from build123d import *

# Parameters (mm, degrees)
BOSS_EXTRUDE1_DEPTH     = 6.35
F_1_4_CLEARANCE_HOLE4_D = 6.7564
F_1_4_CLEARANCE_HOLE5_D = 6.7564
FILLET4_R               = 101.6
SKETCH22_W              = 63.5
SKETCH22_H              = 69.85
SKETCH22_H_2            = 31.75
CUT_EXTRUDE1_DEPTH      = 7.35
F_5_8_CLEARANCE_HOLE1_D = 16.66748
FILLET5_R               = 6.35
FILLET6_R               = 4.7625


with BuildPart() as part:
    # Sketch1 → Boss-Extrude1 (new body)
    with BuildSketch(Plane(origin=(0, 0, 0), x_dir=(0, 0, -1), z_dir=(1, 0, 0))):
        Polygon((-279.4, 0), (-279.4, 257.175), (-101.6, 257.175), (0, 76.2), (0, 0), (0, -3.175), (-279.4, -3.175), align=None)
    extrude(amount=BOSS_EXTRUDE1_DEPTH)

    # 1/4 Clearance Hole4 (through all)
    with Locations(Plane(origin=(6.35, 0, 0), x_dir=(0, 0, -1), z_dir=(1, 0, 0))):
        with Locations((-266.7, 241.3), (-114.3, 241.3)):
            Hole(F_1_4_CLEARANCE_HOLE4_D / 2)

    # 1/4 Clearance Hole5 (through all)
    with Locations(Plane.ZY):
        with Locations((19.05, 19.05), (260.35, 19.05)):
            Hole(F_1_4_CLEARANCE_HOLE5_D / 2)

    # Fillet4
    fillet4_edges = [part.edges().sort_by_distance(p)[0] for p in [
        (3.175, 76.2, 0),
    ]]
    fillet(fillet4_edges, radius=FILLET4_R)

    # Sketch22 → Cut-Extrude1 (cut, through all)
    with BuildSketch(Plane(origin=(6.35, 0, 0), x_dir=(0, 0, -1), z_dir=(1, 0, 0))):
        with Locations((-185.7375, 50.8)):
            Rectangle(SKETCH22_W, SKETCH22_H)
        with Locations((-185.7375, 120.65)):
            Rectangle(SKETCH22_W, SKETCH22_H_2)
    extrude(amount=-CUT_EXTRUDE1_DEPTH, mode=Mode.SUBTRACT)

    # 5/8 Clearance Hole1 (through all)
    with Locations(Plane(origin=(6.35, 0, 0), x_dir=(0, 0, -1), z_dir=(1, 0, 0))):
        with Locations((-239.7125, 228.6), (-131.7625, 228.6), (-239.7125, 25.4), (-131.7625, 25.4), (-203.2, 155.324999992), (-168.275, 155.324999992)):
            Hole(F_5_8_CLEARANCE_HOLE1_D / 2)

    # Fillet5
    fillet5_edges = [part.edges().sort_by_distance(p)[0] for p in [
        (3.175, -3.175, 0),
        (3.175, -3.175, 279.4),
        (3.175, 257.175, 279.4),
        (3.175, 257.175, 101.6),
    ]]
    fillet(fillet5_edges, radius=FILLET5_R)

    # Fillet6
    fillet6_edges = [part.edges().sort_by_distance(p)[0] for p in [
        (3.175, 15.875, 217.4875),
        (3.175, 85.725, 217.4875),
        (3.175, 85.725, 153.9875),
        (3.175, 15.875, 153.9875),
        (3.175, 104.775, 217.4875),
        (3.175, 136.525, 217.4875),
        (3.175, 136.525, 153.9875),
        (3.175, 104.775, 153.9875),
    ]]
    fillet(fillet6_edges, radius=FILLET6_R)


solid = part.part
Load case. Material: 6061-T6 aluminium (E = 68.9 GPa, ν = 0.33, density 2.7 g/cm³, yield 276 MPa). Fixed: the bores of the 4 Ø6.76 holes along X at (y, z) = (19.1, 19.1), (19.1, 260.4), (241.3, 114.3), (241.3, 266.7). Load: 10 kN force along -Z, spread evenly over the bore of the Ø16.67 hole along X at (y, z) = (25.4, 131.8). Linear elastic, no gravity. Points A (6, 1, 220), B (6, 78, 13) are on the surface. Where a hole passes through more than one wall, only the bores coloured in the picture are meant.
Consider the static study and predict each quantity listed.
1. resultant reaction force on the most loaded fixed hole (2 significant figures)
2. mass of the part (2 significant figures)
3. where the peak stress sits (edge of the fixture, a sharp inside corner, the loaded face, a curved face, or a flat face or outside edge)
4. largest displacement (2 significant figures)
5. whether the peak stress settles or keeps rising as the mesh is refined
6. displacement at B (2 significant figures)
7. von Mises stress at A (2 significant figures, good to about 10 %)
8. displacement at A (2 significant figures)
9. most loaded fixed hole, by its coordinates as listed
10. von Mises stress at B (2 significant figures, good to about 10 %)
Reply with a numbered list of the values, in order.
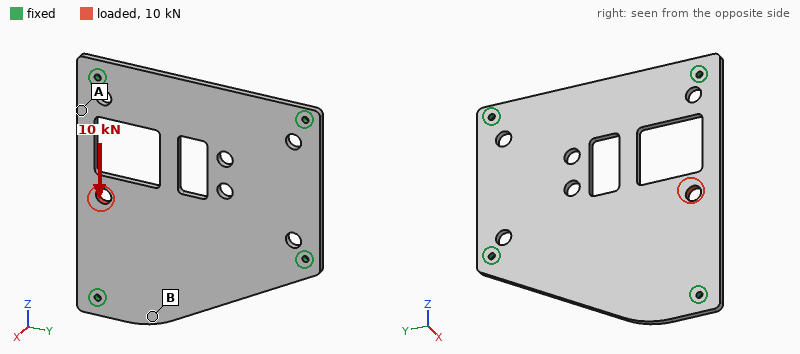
1. 6.2 kN
2. 950 g
3. edge of the fixture
4. 47 µm
5. keeps rising
6. 16 µm
7. 18 MPa
8. 15 µm
9. (19.1, 19.1)
10. 6.3 MPa
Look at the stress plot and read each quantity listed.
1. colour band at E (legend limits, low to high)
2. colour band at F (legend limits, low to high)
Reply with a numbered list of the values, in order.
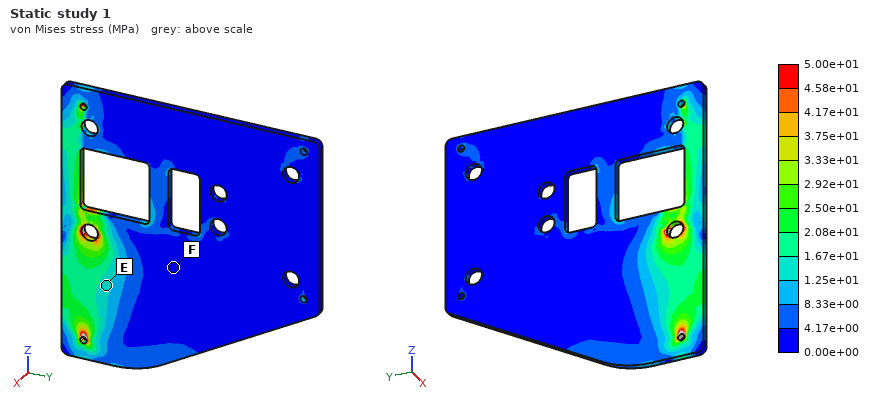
1. 1.25e+01 to 1.67e+01 MPa
2. 0.00e+00 to 4.17e+00 MPa
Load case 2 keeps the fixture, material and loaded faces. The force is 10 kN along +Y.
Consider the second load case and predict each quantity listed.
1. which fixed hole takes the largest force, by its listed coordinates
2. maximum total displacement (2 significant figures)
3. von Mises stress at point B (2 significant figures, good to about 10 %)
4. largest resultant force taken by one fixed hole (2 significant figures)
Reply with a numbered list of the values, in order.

1. (241.3, 114.3)
2. 81 µm
3. 9.0 MPa
4. 6.0 kN
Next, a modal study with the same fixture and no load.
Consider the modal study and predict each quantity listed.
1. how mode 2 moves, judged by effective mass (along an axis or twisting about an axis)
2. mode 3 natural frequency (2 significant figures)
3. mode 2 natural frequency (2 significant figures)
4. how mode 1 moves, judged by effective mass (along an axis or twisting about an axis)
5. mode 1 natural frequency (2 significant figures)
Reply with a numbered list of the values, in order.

1. twisting about Y
2. 650 Hz
3. 620 Hz
4. along X
5. 420 Hz
